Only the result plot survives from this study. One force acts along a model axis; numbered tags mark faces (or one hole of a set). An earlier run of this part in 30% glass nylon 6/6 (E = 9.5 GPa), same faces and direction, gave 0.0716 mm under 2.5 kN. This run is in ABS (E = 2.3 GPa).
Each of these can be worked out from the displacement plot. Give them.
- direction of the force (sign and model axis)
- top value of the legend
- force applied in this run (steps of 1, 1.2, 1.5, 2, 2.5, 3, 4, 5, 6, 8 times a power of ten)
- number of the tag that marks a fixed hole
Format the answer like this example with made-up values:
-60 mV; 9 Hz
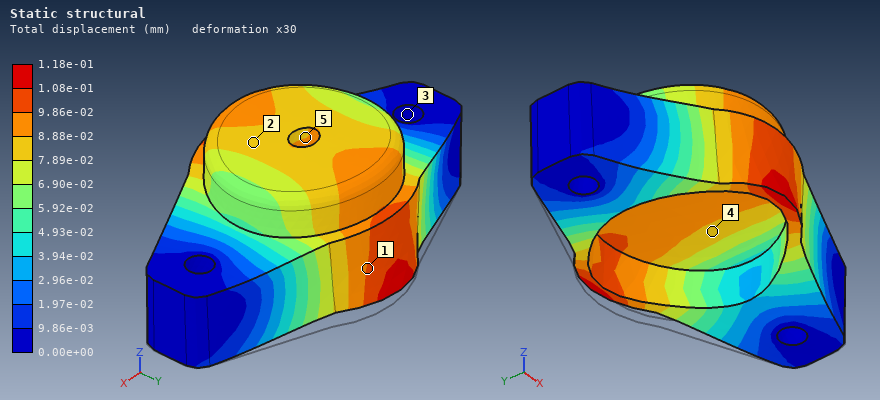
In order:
+Z; 1.18e-01 mm; 1 kN; 3
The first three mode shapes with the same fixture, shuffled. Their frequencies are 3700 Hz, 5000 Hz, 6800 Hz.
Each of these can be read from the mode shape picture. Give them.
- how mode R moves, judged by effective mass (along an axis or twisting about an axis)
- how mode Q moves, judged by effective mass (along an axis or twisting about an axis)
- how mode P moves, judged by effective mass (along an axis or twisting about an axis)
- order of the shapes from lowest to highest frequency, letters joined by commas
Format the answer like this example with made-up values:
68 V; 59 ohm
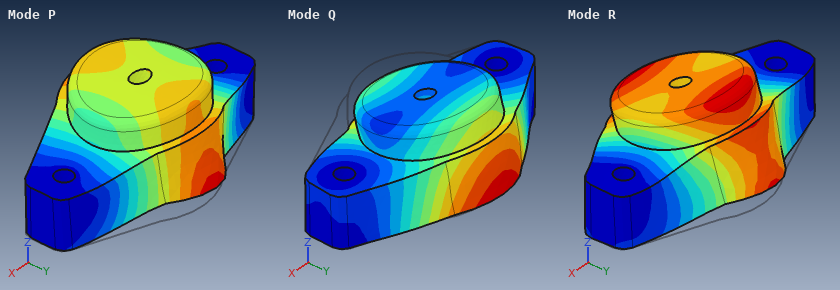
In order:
along Y; along Y; along Z; R, P, Q
